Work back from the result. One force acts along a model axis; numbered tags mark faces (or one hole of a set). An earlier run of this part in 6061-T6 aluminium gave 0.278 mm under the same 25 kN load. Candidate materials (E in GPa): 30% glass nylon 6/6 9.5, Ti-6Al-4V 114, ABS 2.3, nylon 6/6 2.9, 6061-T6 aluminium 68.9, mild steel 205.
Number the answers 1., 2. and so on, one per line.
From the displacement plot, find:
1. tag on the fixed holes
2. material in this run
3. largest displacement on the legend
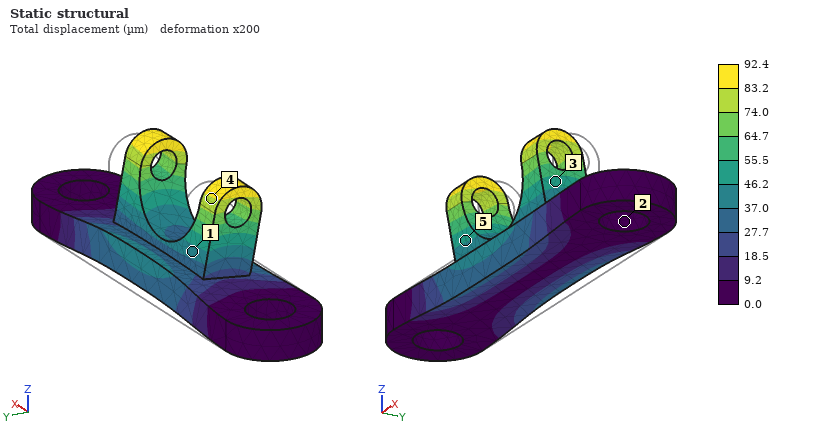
1. 2
2. mild steel
3. 92.4 µm
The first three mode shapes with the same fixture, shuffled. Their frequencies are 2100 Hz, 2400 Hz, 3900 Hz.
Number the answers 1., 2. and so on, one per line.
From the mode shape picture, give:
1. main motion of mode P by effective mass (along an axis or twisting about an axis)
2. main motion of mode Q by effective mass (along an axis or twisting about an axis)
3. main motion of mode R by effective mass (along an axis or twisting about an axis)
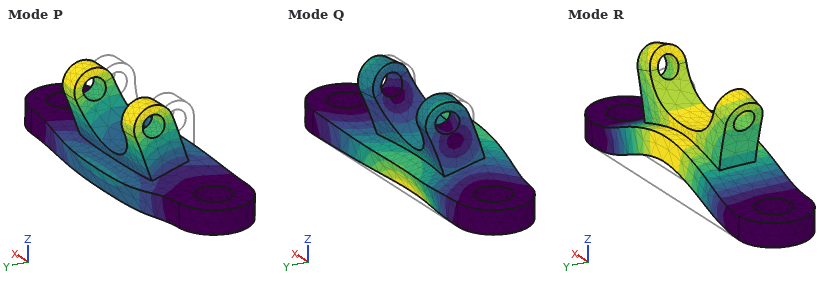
1. along Y
2. along Y
3. along Z
